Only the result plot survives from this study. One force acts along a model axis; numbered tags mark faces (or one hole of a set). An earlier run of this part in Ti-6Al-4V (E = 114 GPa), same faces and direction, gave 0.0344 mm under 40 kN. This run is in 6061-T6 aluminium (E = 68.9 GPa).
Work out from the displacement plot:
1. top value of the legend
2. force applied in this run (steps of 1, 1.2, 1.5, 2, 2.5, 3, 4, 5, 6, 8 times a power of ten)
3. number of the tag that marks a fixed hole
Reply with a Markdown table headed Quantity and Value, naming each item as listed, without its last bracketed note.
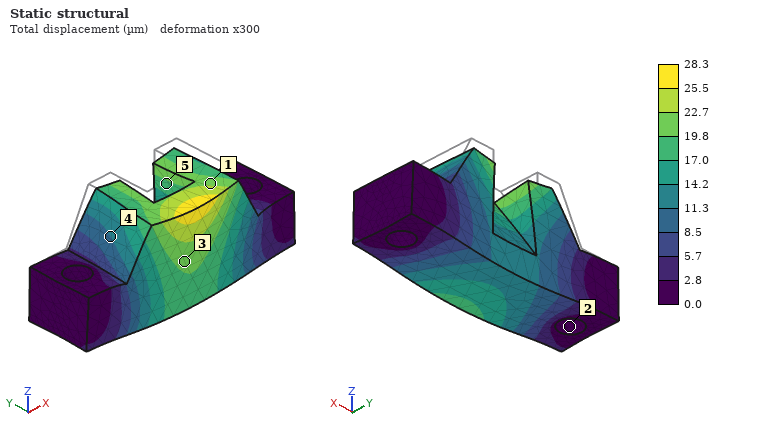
| Quantity | Value |
|---|---|
| top value of the legend | 28.3 µm |
| force applied in this run | 20 kN |
| number of the tag that marks a fixed hole | 2 |
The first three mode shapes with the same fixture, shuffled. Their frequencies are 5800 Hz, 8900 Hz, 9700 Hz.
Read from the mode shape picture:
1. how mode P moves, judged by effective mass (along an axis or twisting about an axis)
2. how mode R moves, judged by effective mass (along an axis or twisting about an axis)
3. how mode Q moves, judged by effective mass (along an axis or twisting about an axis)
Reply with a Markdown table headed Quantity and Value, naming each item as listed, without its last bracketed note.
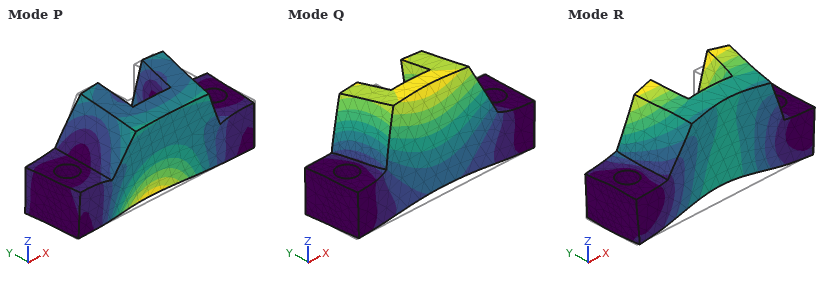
| Quantity | Value |
|---|---|
| how mode P moves, judged by effective mass | along Y |
| how mode R moves, judged by effective mass | along Z |
| how mode Q moves, judged by effective mass | along Y |
